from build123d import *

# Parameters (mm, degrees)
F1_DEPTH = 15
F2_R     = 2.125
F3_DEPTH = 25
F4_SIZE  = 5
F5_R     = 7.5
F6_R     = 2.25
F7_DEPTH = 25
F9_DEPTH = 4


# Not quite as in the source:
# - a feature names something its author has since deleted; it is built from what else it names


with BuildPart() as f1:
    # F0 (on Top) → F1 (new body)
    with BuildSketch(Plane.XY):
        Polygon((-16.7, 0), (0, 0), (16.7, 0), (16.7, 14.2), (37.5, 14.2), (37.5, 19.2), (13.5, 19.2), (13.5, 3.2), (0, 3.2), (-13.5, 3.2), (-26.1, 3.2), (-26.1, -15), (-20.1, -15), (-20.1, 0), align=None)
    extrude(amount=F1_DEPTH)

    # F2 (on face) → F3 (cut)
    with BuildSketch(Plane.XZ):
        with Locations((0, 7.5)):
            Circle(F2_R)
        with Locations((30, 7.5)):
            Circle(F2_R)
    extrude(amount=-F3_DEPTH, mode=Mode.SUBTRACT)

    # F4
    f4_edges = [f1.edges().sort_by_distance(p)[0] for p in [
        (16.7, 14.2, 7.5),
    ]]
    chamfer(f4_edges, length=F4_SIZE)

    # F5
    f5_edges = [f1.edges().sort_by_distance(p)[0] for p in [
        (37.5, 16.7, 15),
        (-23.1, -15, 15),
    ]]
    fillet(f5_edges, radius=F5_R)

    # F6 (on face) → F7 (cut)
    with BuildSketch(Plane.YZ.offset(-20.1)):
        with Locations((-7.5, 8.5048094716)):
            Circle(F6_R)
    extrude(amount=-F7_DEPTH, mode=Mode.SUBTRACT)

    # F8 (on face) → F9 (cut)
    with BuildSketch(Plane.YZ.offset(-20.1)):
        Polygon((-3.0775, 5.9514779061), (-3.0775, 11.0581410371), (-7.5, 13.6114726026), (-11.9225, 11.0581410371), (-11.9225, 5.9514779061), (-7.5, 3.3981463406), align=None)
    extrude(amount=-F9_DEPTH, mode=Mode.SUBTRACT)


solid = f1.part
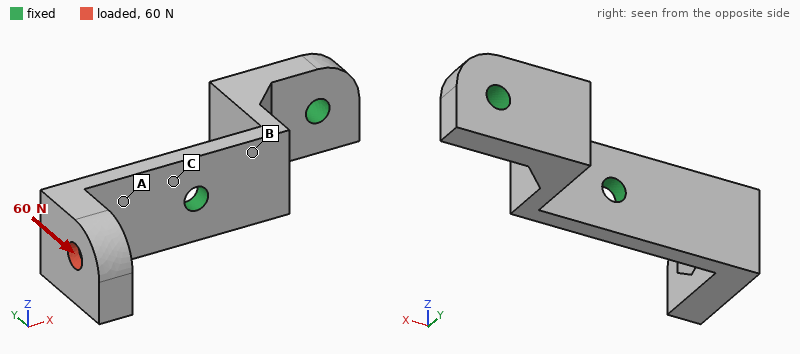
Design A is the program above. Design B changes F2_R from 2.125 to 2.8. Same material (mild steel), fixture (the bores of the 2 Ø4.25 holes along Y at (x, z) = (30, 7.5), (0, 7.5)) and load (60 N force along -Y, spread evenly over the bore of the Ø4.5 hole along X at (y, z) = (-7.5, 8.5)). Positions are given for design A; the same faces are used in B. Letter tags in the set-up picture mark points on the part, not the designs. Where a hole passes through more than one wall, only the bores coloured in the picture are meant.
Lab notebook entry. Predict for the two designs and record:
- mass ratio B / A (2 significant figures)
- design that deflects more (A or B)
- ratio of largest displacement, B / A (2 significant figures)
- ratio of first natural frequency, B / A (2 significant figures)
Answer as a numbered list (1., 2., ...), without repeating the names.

1. 0.98
2. A
3. 0.91
4. 1.1
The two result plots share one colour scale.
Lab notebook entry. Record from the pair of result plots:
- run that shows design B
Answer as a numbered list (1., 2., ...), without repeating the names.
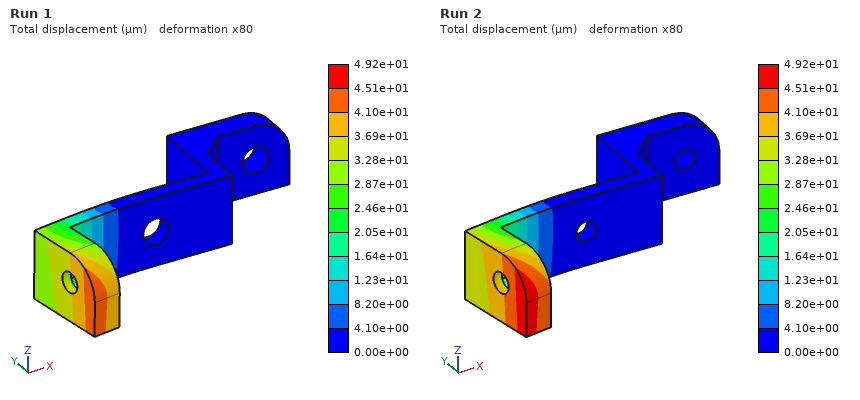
1. Run 1
